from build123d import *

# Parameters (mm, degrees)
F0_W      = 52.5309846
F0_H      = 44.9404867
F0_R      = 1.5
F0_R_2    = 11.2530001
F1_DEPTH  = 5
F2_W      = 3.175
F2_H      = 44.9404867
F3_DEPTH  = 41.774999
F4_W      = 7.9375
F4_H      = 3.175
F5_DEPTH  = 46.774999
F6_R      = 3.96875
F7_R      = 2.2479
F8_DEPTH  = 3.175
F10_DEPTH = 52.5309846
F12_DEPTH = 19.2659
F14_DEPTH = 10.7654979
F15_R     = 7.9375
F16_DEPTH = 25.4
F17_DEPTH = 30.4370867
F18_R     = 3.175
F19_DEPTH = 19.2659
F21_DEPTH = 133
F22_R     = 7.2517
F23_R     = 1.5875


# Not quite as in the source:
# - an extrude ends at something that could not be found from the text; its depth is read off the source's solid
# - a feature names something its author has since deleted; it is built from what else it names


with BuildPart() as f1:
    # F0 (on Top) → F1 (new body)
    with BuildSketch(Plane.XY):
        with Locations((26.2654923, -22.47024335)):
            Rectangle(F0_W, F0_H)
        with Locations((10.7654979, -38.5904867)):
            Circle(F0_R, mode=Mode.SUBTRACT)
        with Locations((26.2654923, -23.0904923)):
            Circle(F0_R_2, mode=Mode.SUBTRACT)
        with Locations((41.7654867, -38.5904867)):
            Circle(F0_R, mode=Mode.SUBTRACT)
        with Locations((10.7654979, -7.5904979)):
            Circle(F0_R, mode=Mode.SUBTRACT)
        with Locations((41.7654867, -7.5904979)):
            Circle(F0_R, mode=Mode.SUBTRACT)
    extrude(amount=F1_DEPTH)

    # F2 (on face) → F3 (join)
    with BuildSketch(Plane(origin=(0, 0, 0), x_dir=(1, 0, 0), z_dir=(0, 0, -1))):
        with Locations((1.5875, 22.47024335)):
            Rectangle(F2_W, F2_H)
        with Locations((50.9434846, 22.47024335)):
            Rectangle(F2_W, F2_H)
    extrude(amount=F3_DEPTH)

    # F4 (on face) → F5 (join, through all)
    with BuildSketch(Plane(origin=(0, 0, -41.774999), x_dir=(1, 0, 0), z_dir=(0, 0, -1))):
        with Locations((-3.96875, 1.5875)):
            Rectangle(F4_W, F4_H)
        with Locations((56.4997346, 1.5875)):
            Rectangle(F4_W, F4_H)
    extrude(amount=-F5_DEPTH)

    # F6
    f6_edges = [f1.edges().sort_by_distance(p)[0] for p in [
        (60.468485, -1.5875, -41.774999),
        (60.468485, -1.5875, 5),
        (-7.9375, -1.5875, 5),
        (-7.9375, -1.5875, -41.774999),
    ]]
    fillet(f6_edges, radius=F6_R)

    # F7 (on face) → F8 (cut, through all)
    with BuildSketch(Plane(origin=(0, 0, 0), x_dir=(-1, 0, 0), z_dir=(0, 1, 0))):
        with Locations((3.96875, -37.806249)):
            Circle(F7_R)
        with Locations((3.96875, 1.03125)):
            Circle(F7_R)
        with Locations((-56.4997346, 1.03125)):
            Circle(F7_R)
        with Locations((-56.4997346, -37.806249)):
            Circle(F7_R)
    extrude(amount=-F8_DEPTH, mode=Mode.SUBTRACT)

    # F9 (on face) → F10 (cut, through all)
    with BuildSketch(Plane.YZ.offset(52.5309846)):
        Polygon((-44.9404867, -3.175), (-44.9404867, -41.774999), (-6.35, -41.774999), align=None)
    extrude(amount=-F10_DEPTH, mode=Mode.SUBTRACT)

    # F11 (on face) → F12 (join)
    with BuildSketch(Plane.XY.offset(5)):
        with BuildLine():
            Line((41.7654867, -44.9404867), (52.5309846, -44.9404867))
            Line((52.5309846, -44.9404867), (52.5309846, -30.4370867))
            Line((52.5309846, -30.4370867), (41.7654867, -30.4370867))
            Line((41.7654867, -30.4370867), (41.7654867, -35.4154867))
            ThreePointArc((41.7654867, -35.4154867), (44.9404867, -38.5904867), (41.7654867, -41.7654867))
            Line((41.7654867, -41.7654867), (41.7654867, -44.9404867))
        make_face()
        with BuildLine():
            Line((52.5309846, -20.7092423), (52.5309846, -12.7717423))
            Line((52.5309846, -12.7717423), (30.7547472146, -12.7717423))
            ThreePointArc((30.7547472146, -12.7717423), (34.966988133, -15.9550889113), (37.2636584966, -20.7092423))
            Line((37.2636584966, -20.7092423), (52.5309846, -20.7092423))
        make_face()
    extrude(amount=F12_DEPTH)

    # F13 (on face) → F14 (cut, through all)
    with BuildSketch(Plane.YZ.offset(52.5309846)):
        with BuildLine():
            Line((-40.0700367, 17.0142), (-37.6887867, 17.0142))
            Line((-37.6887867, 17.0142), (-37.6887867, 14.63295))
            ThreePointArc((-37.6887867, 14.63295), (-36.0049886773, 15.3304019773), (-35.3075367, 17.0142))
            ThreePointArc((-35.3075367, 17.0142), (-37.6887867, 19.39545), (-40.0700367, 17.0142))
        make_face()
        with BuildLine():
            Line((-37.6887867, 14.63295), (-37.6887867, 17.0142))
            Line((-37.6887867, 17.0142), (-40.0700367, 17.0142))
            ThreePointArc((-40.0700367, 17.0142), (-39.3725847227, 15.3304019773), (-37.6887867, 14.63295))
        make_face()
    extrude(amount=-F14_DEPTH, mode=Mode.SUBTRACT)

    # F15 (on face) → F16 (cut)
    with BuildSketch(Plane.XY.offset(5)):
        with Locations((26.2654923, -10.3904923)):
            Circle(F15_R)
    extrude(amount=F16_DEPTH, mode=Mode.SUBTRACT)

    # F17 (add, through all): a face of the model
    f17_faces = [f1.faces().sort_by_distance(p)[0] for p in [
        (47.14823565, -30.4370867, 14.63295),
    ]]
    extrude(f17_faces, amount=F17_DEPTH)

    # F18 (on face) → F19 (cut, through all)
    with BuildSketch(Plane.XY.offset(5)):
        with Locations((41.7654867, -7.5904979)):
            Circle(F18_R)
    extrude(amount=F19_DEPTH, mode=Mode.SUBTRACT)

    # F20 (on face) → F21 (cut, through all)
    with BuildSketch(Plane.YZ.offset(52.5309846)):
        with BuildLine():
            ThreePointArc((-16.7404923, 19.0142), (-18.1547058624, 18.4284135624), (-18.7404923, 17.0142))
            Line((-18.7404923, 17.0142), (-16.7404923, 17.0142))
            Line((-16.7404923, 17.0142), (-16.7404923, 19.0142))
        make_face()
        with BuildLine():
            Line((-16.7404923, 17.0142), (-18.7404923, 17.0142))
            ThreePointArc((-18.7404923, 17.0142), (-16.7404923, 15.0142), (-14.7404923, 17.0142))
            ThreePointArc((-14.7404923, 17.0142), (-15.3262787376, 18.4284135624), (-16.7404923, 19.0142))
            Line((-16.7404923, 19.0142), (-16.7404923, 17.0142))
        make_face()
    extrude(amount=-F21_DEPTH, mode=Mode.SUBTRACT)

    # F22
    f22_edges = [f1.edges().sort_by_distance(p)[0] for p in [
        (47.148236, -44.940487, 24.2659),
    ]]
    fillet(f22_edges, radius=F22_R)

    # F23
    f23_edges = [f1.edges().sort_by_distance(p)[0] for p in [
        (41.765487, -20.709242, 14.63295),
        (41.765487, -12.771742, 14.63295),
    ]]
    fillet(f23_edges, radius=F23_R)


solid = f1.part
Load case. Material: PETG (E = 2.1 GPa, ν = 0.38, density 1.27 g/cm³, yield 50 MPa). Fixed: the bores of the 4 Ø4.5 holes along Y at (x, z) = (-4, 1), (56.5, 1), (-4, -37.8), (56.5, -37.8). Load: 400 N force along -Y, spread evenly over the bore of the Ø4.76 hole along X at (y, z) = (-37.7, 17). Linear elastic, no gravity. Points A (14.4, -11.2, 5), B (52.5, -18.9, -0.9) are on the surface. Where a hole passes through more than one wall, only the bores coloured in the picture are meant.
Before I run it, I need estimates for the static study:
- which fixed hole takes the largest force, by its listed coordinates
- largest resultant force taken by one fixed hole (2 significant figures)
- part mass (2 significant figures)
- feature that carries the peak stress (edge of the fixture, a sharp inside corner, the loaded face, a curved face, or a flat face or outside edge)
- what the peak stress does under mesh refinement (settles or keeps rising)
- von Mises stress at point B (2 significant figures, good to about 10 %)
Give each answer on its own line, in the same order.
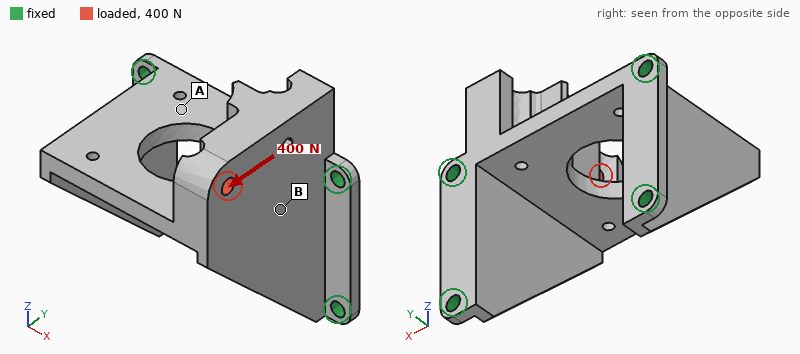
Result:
(56.5, 1)
520 N
36 g
edge of the fixture
keeps rising
4.5 MPa
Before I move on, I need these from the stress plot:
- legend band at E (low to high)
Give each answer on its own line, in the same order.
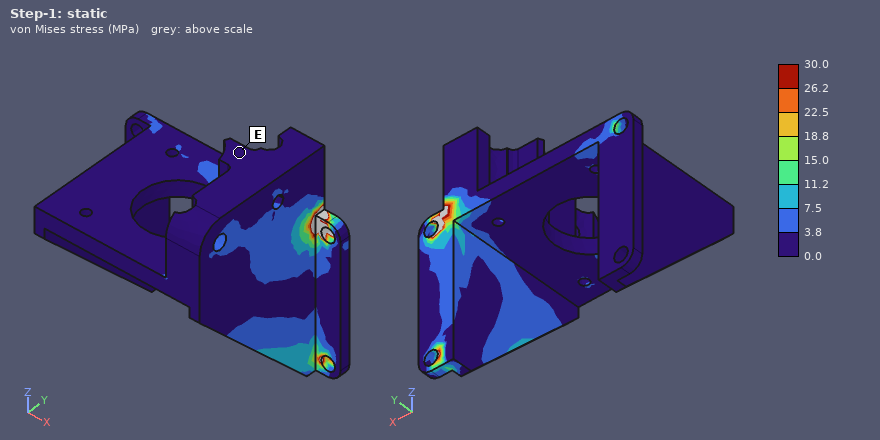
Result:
0.0 to 3.8 MPa
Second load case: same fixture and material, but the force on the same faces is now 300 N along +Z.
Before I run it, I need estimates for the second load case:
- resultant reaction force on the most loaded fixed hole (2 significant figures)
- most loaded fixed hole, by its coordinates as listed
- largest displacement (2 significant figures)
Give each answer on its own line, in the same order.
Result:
340 N
(56.5, -37.8)
0.67 mm
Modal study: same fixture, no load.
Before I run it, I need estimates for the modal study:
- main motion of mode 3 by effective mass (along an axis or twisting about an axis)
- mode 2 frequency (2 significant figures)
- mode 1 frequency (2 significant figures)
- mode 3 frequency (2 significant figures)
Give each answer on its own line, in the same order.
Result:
along X
1100 Hz
890 Hz
1500 Hz
